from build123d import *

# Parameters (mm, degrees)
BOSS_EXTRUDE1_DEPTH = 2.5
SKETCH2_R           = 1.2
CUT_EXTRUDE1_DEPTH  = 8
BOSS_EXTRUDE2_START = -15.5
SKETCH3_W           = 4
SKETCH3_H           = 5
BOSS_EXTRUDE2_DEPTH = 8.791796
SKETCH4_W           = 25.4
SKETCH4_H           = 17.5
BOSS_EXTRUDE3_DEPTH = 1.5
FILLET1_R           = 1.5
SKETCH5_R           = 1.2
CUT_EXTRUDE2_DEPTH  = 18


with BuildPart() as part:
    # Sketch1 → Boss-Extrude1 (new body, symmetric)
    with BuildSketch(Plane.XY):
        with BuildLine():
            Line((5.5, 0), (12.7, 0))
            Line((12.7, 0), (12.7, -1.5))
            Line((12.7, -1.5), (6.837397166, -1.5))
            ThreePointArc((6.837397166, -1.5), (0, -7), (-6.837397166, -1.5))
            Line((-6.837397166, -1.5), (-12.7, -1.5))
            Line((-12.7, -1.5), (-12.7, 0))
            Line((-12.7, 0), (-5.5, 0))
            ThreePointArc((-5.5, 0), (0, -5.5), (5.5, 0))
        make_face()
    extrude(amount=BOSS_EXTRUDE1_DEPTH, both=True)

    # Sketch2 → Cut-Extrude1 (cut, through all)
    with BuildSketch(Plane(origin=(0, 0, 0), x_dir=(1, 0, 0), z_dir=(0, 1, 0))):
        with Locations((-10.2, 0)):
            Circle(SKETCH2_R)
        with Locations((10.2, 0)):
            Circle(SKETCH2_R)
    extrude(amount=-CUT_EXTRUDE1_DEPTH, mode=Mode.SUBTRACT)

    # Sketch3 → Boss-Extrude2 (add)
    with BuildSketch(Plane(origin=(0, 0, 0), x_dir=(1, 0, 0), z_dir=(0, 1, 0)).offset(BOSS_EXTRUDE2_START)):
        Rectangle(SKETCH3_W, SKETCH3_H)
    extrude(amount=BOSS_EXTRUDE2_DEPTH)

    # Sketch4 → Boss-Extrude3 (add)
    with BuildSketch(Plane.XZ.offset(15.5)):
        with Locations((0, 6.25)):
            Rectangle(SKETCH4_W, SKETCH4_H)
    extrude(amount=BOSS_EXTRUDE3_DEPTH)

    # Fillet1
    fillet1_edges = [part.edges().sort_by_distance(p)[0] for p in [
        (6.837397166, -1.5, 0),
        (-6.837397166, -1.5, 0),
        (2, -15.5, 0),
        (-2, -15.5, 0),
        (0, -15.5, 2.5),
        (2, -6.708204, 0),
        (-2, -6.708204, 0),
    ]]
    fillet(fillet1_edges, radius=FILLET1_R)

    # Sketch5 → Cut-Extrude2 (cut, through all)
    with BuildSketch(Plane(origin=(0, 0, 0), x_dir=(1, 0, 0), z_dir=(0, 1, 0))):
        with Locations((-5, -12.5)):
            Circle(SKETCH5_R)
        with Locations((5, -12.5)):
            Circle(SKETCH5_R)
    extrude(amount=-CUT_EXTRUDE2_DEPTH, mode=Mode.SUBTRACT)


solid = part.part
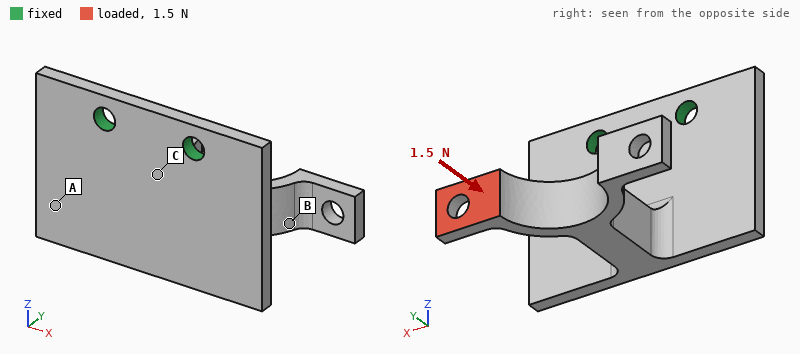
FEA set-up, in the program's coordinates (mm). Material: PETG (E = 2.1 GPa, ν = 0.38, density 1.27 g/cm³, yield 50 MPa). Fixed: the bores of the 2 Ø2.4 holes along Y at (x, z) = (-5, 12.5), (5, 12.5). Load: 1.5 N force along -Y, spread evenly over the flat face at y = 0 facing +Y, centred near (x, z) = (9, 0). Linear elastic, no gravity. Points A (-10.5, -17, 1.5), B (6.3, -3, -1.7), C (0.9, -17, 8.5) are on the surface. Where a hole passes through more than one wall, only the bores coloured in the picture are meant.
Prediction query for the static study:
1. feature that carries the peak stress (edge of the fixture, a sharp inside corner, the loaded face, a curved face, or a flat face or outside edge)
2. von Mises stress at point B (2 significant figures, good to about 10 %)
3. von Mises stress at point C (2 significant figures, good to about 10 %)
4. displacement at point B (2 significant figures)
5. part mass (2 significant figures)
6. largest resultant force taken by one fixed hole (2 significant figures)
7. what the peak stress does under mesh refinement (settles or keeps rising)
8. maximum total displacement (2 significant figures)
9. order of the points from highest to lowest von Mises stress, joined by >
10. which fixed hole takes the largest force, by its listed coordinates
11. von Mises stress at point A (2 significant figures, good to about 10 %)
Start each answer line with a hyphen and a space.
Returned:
- edge of the fixture
- 2.7 MPa
- 1.7 MPa
- 0.22 mm
- 1.3 g
- 1.9 N
- keeps rising
- 0.40 mm
- B > C > A
- (5, 12.5)
- 0.64 MPa
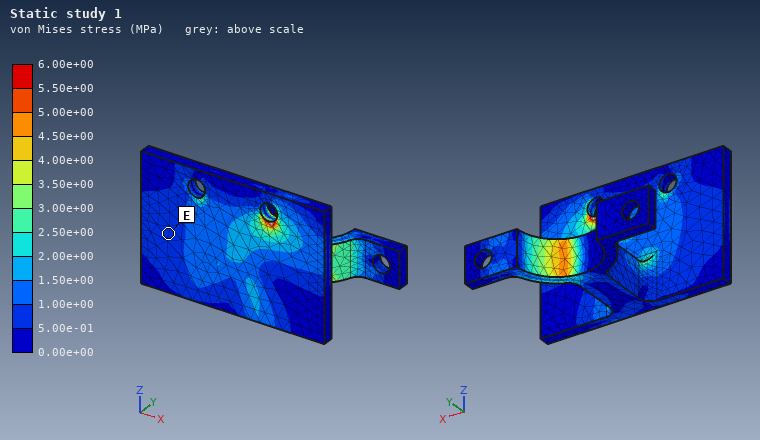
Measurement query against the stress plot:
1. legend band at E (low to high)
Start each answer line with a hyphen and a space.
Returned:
- 5.00e-01 to 1.00e+00 MPa
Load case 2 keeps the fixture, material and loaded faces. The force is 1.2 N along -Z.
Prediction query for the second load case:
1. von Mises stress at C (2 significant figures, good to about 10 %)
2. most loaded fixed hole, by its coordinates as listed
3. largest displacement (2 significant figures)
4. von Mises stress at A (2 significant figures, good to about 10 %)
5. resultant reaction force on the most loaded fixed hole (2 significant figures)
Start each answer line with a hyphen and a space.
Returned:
- 1.9 MPa
- (5, 12.5)
- 0.35 mm
- 0.96 MPa
- 1.6 N
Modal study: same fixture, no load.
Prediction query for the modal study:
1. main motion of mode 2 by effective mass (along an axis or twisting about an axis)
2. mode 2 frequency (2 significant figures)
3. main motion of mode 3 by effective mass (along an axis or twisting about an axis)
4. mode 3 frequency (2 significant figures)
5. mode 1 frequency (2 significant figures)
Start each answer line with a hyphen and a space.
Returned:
- along X
- 820 Hz
- along Y
- 1800 Hz
- 570 Hz
